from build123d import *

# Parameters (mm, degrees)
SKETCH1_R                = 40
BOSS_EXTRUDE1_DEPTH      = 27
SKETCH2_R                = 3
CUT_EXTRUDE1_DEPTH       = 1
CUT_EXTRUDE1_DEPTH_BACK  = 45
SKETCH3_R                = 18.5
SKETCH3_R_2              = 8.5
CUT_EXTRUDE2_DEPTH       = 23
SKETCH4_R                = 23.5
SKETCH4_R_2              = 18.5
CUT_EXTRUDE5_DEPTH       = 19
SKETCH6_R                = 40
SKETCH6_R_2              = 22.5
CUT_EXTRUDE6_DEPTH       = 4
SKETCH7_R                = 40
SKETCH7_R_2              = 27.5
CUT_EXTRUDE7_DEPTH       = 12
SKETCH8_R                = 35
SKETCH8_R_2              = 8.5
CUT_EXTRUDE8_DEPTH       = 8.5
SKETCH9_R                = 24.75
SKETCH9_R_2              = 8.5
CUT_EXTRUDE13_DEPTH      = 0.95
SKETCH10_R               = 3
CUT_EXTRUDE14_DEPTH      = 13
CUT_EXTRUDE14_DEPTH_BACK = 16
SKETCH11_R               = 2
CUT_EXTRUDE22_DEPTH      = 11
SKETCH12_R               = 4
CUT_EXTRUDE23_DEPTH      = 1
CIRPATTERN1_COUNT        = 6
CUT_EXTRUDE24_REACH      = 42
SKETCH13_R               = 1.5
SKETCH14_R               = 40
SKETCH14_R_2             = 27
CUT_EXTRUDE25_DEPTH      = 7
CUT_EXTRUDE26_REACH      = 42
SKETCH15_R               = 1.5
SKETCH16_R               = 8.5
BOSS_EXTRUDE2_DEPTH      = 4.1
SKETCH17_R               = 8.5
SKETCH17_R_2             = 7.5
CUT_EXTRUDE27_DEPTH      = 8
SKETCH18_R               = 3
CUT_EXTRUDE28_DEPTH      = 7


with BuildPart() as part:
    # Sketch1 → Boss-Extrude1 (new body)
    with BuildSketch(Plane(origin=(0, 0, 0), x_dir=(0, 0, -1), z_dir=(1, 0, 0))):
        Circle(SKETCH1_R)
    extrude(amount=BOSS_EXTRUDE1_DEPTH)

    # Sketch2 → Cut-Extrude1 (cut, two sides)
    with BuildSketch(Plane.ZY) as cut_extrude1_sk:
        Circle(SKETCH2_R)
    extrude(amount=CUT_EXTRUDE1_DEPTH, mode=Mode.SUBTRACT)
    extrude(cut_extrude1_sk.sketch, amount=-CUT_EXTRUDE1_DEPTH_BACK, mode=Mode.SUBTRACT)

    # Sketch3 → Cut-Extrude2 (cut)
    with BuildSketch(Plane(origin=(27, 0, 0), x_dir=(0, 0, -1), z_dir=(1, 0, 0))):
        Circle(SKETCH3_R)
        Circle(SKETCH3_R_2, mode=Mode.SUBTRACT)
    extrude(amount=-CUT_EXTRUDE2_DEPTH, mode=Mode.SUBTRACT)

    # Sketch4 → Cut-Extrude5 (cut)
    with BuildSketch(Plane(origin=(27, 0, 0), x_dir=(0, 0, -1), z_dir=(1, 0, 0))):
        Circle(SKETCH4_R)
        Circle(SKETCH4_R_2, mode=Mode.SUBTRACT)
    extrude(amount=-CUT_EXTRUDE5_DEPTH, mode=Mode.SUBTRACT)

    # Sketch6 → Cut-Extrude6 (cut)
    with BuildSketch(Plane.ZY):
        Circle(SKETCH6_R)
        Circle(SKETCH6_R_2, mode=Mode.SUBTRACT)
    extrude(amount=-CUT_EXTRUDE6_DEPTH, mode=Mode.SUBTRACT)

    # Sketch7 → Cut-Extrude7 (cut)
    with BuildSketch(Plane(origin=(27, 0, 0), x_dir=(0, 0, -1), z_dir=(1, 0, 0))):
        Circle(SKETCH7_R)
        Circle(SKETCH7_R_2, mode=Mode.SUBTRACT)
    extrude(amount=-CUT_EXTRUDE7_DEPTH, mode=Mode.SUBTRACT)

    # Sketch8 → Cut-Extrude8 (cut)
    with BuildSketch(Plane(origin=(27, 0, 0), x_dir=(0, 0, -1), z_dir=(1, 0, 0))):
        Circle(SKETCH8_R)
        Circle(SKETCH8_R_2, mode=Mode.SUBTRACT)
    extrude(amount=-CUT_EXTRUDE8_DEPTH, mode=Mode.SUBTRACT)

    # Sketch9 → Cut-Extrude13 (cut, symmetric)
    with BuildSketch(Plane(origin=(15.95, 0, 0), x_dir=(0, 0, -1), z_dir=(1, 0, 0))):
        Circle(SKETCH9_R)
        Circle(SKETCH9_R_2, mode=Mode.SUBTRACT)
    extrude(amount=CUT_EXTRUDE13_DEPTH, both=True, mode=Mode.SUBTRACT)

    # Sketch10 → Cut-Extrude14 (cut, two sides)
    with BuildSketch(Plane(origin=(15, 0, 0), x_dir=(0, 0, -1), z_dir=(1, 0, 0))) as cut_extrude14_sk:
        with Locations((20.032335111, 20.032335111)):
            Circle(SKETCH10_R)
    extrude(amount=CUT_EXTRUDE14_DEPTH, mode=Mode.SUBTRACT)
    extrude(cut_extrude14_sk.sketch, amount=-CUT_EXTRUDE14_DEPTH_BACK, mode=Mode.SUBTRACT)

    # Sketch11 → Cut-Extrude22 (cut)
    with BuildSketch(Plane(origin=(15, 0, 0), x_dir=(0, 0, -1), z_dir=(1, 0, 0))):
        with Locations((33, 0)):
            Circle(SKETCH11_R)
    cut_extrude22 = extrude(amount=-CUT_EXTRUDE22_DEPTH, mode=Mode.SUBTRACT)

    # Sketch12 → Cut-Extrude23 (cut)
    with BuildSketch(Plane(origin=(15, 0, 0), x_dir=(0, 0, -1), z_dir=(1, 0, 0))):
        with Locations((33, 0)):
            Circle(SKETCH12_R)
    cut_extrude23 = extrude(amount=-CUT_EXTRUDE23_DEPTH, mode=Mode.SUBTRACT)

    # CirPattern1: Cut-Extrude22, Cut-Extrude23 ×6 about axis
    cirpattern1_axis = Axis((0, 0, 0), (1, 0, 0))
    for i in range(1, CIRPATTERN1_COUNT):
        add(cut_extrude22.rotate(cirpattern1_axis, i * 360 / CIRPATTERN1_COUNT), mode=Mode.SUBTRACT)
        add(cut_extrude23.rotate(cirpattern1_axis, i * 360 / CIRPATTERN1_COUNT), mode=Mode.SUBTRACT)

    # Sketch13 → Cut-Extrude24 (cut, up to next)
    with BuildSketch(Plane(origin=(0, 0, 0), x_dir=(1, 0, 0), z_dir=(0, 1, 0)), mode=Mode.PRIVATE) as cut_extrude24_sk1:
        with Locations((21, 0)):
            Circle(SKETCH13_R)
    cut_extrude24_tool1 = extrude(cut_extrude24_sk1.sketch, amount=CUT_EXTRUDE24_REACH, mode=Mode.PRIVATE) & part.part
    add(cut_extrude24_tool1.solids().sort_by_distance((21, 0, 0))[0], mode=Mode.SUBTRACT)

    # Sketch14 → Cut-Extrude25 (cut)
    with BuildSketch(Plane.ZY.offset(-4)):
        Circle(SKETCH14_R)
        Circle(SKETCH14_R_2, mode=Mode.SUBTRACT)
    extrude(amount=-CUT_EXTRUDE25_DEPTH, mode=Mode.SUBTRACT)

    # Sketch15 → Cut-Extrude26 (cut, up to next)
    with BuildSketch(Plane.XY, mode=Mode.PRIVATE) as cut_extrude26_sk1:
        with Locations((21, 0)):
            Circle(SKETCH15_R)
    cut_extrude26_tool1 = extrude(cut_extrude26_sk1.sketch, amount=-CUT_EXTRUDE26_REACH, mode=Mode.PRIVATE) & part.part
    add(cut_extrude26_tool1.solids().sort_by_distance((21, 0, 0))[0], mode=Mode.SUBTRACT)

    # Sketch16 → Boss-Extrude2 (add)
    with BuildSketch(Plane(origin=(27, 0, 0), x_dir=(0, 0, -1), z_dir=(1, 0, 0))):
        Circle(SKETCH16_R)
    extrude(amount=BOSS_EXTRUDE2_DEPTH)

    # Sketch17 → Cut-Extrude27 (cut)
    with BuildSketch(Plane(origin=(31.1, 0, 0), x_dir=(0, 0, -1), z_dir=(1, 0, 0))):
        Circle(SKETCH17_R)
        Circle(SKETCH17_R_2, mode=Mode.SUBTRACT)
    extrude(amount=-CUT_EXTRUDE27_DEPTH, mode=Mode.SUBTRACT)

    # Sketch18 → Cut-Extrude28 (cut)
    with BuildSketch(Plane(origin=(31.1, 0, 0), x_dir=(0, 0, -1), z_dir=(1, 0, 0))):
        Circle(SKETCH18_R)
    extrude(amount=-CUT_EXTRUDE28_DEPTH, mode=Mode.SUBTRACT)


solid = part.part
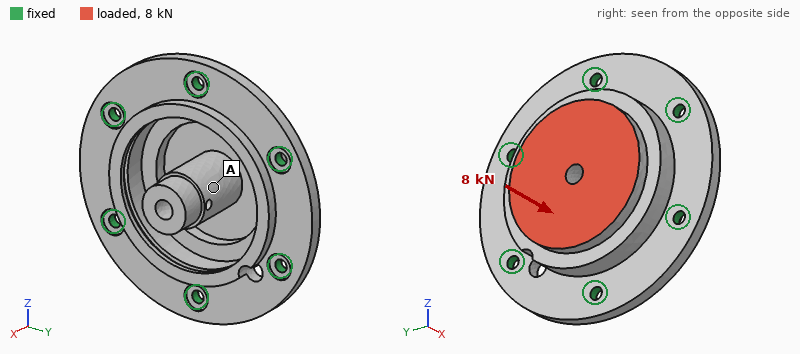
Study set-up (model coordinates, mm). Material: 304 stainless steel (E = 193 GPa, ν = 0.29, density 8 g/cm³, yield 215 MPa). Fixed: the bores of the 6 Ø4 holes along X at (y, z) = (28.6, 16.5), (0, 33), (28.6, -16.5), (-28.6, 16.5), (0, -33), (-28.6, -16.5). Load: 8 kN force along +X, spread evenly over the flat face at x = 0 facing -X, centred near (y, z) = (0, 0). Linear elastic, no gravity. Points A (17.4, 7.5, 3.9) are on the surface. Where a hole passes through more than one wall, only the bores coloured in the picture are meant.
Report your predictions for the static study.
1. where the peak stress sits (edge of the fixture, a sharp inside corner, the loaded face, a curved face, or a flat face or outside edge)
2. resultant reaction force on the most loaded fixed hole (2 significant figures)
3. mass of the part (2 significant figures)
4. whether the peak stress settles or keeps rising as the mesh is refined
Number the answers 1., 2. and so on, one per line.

1. edge of the fixture
2. 1.6 kN
3. 260 g
4. keeps rising
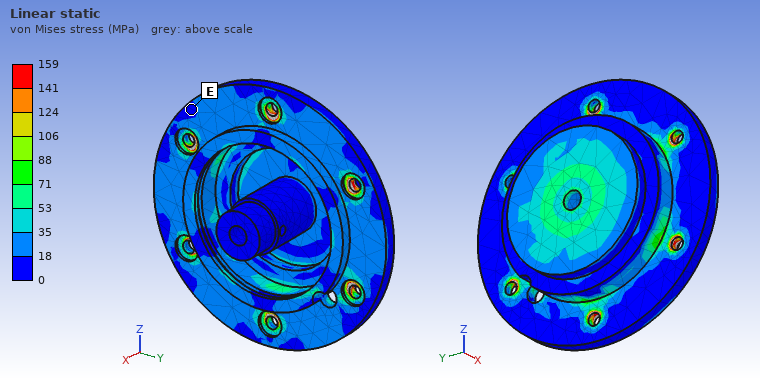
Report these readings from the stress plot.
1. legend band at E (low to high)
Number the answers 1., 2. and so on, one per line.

1. 0 to 18 MPa
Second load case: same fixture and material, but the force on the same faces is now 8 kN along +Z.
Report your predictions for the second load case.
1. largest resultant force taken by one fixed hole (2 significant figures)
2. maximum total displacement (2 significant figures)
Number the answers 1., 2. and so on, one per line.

1. 1.8 kN
2. 14 µm
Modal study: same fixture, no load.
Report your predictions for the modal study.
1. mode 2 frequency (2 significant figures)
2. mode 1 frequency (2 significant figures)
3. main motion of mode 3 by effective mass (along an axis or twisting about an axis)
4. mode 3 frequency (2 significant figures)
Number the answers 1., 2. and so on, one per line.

1. 6300 Hz
2. 6300 Hz
3. along X
4. 8800 Hz
